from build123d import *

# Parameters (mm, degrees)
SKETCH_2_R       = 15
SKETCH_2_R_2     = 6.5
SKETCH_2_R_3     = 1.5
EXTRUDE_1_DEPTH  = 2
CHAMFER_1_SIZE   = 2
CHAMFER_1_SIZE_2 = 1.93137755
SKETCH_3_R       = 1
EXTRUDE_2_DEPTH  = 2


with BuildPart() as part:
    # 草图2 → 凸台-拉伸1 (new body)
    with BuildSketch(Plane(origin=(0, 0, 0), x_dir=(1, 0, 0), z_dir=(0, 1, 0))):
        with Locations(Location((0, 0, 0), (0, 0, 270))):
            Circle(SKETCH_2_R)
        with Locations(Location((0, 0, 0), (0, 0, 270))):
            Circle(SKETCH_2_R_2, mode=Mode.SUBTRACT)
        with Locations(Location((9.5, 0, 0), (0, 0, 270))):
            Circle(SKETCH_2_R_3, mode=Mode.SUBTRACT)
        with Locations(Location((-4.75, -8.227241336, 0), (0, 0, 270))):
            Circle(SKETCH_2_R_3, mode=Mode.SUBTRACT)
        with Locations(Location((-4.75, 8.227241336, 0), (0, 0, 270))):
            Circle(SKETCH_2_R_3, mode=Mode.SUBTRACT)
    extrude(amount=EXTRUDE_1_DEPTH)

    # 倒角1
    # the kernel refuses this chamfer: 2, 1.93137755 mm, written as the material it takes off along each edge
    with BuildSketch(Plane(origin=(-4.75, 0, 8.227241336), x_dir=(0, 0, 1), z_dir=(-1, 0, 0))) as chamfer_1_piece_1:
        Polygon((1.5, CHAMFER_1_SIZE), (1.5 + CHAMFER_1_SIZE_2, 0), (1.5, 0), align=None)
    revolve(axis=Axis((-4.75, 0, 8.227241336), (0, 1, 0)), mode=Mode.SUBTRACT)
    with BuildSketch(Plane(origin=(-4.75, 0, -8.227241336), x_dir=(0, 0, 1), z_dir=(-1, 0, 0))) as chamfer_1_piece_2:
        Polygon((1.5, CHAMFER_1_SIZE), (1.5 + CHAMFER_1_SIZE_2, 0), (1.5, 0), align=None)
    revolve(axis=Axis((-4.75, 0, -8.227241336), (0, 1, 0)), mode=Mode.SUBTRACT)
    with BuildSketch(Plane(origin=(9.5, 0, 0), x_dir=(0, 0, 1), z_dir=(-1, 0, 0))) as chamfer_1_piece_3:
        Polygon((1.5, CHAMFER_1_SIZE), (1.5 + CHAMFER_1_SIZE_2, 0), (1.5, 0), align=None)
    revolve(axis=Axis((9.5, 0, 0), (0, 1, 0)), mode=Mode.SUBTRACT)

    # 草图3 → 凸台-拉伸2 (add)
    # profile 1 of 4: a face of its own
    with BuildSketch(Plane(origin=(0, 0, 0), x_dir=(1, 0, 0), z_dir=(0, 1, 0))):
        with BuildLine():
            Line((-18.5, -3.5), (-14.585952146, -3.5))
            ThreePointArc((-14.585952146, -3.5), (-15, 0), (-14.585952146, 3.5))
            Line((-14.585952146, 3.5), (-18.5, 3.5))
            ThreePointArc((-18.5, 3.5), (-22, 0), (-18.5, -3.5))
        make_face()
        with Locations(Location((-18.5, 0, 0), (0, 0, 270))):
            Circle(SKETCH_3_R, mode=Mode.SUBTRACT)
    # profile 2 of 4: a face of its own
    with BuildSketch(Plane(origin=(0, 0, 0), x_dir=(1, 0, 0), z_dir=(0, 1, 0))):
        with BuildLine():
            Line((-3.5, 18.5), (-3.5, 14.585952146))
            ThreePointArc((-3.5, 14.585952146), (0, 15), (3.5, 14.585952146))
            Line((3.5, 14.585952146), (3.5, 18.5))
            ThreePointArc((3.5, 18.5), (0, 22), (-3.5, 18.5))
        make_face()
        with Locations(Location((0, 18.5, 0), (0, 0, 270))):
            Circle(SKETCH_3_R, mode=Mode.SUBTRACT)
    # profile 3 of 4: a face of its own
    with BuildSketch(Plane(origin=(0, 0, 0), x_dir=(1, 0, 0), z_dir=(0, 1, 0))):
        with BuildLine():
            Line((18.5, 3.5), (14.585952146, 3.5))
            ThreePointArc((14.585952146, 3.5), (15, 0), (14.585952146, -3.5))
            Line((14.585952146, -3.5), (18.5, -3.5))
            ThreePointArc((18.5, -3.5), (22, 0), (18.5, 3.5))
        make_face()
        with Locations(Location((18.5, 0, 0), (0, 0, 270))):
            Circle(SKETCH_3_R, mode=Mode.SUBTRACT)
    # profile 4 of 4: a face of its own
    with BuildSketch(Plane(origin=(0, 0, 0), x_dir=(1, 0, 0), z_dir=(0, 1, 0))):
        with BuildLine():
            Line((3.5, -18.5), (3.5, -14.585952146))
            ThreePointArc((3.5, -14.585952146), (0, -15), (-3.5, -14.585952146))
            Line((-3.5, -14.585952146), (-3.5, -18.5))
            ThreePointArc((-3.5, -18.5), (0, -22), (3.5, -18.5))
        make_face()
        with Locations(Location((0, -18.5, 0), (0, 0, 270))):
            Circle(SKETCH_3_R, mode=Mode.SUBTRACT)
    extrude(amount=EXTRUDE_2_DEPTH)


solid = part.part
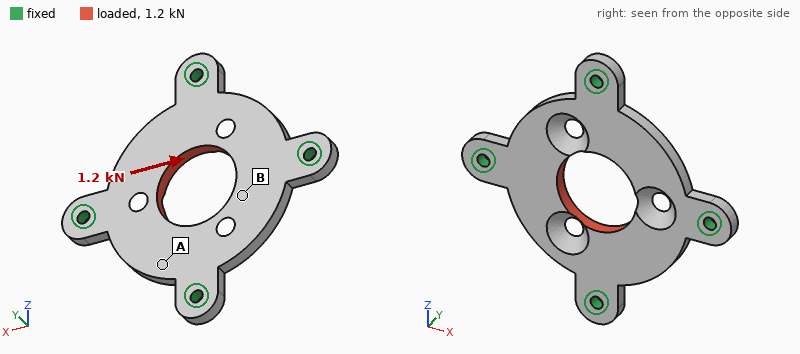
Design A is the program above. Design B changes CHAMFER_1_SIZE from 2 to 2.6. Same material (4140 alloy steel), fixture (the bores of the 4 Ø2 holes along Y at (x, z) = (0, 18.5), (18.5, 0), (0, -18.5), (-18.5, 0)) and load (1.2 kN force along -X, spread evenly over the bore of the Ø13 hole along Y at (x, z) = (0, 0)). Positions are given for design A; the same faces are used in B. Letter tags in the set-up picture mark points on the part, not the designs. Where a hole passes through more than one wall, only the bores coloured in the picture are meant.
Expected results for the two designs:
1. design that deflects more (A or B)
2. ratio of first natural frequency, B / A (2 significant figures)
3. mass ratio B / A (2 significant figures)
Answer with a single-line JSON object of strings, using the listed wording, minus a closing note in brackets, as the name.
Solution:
{"design that deflects more": "B", "ratio of first natural frequency, B / A": "1.0", "mass ratio B / A": "0.99"}
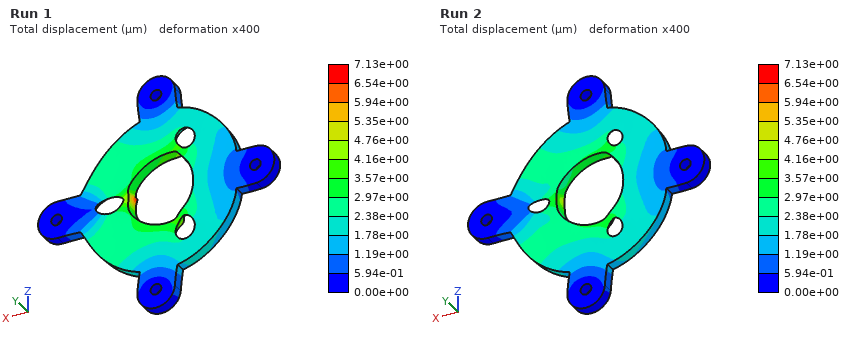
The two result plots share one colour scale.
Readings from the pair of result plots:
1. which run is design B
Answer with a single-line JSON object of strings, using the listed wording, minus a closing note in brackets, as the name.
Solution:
{"which run is design B": "Run 1"}
